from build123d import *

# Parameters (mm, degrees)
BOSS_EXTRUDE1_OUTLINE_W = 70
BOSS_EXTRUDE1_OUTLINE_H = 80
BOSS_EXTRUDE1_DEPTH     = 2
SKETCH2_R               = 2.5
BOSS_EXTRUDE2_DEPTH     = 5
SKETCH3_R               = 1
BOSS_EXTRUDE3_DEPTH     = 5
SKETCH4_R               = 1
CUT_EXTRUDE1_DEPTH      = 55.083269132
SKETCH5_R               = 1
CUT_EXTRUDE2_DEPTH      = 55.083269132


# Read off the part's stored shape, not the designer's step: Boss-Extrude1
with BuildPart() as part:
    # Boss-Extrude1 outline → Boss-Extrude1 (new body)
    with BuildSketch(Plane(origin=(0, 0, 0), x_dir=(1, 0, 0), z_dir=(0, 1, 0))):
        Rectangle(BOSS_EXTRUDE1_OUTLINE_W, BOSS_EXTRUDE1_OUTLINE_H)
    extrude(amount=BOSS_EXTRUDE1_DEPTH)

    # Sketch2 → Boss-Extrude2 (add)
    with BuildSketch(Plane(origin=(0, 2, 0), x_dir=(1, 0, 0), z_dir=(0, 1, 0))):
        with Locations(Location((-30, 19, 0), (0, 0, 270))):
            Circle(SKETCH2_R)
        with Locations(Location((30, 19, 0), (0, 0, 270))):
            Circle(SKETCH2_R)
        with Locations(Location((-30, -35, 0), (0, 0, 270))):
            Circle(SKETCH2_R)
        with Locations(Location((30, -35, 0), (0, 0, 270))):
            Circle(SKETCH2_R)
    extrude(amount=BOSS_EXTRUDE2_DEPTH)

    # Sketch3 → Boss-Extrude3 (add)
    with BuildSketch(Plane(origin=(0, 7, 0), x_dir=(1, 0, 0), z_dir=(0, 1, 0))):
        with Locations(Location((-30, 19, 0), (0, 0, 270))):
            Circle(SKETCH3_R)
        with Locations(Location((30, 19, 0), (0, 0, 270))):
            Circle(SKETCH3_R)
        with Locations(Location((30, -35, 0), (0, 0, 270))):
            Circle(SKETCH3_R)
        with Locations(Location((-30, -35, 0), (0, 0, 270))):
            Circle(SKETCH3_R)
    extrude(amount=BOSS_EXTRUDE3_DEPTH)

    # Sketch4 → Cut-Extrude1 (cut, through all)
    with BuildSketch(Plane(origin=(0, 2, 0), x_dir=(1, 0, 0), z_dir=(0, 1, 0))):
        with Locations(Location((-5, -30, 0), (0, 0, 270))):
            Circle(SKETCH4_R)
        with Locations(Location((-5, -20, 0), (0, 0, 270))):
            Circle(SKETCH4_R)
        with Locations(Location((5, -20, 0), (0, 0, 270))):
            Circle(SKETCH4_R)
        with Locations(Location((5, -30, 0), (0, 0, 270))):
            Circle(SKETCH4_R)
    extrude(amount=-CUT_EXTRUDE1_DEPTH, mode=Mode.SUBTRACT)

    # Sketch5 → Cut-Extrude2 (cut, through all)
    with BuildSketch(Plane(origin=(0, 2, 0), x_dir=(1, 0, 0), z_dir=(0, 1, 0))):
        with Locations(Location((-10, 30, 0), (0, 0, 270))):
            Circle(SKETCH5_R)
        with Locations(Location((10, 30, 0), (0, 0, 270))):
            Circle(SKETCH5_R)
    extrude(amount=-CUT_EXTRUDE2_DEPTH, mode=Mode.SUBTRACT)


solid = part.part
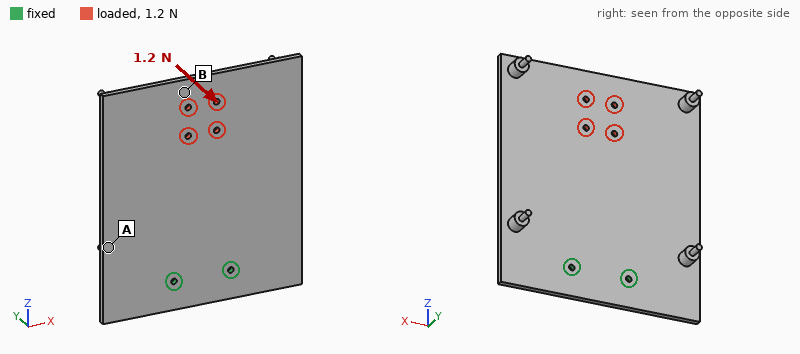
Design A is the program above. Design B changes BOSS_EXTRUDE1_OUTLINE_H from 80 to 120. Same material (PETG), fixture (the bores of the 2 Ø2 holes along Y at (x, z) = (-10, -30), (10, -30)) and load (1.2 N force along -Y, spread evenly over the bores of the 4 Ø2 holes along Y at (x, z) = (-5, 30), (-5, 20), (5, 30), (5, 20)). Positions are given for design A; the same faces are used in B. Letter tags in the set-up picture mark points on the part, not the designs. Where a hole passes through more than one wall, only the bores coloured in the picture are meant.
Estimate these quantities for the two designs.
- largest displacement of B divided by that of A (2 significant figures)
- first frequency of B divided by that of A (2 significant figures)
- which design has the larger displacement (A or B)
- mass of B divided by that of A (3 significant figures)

1.3
0.64
B
1.48
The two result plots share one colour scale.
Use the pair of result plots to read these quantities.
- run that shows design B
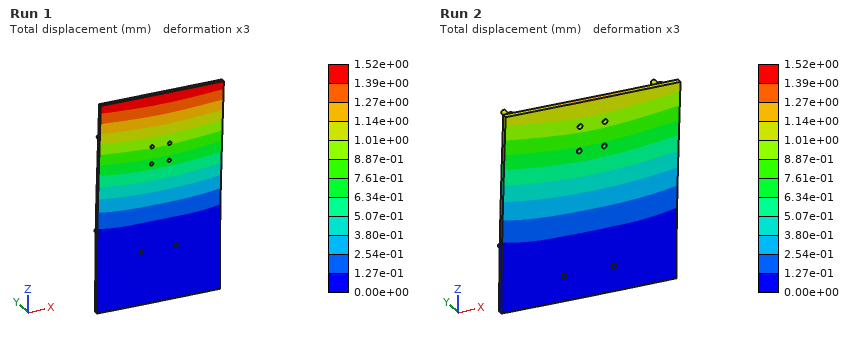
Run 1
